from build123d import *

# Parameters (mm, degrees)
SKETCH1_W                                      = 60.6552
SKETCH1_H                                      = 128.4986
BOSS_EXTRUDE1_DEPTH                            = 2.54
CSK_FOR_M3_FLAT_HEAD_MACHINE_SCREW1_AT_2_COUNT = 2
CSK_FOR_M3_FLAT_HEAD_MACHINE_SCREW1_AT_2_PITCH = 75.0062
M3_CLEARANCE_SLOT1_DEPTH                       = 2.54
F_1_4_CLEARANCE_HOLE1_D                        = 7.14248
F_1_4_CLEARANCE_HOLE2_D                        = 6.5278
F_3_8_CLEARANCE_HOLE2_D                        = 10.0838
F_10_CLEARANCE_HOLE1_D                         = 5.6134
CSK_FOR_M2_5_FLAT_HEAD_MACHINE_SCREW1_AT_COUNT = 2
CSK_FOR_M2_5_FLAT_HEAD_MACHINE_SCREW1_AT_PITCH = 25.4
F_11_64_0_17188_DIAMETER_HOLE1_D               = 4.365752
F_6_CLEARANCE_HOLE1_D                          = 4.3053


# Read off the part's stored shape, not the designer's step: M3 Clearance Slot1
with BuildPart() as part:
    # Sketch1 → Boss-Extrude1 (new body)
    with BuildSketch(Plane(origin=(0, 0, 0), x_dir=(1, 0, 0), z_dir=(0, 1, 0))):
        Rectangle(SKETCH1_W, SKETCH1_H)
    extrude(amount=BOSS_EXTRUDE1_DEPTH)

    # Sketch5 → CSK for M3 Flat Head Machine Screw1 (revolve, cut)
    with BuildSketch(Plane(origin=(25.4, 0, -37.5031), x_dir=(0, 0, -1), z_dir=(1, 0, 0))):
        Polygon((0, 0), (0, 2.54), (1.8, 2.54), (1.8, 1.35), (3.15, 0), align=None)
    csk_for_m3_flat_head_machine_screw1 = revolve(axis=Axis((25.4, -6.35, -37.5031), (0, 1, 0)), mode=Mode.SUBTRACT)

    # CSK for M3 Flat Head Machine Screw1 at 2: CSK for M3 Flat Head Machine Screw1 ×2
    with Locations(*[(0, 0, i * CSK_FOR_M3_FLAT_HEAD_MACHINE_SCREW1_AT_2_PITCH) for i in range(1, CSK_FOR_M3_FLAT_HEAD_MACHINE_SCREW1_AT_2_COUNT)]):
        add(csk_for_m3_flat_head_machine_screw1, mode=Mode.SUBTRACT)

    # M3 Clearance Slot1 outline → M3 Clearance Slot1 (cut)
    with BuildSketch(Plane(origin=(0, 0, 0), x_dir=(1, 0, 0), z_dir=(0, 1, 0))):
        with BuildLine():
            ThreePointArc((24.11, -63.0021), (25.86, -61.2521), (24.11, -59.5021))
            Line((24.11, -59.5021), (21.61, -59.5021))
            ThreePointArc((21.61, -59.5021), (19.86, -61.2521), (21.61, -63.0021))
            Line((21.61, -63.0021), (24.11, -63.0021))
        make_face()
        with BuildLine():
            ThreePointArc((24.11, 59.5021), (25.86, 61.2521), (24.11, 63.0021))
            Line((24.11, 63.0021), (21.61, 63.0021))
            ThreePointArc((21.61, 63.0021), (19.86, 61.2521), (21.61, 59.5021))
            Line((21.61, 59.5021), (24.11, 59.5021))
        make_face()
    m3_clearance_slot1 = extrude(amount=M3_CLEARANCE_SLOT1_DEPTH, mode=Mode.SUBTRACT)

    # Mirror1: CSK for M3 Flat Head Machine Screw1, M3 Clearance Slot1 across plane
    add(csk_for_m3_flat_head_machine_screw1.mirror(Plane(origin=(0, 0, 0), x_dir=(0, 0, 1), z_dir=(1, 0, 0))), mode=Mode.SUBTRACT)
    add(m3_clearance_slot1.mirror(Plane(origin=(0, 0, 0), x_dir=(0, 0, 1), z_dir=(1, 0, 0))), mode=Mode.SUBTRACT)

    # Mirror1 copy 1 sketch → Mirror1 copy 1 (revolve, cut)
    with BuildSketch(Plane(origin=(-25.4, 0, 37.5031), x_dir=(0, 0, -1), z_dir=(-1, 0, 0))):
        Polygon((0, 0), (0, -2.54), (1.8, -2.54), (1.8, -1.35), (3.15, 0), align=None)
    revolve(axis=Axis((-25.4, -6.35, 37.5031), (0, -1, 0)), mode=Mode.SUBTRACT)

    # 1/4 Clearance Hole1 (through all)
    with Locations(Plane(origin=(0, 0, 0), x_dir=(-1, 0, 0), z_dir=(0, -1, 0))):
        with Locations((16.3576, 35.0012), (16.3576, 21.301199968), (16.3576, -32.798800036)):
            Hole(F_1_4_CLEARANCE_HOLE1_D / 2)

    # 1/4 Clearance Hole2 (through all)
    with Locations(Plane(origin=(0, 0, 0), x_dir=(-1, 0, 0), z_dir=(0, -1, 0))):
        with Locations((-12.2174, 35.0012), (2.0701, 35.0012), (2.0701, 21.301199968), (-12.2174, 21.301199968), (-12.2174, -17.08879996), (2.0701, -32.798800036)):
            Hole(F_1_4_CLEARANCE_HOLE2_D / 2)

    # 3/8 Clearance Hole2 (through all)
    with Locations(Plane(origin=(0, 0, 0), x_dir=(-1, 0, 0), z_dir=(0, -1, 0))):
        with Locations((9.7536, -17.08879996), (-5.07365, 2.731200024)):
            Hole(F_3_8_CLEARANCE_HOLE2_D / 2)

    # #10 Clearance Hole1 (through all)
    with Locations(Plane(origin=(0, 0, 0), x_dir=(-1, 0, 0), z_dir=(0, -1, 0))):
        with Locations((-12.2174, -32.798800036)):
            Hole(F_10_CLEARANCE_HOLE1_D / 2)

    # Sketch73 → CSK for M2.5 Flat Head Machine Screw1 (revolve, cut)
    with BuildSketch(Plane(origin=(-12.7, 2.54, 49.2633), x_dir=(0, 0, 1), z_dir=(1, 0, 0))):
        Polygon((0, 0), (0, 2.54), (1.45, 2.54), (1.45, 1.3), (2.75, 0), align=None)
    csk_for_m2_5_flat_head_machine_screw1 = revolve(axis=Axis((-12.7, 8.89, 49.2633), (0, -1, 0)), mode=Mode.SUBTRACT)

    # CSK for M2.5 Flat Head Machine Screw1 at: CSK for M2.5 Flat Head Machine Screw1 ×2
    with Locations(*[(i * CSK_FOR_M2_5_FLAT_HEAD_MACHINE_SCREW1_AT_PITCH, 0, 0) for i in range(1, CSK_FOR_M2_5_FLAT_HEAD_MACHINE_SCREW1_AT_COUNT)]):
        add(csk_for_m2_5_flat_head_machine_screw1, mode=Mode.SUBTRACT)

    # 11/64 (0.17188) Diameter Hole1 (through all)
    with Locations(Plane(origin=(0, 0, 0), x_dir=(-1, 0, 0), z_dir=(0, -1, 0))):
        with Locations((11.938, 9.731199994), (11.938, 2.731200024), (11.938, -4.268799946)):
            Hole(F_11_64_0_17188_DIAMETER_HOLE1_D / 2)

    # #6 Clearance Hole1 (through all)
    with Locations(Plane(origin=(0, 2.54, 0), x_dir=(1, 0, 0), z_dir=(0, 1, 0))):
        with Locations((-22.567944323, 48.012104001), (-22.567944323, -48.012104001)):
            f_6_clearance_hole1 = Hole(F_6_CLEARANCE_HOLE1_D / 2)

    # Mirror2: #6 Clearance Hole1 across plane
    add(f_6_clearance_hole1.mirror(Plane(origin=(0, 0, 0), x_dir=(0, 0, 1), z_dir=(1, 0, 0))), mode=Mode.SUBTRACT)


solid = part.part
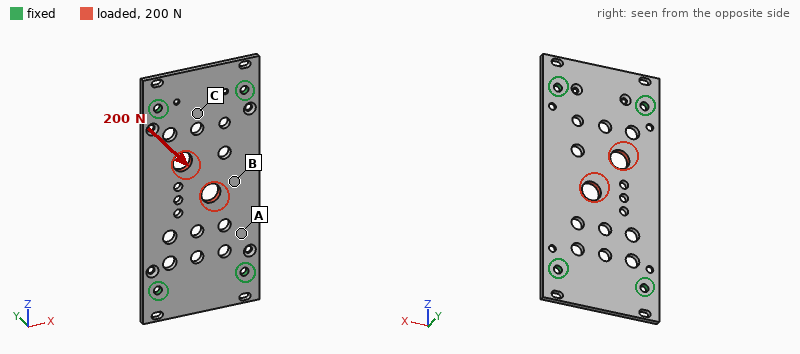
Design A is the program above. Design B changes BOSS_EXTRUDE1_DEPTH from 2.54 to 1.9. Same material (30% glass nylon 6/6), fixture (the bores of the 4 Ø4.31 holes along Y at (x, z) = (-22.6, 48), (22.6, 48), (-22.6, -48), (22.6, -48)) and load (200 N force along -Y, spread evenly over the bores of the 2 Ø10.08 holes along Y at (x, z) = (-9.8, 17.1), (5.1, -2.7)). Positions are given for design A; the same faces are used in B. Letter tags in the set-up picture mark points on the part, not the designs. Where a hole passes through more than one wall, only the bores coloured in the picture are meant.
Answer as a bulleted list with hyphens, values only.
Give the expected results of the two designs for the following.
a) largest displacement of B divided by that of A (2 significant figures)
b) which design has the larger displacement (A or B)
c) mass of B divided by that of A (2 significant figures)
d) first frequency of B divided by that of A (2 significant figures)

- 2.3
- B
- 0.75
- 0.76
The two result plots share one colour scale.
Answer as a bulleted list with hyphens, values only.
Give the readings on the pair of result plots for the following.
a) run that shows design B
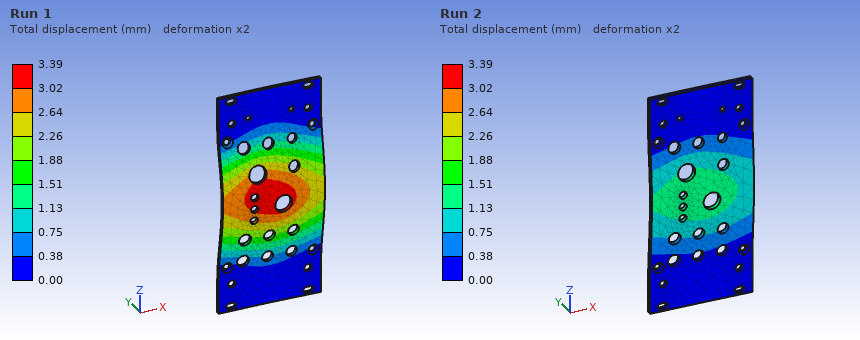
- Run 1
